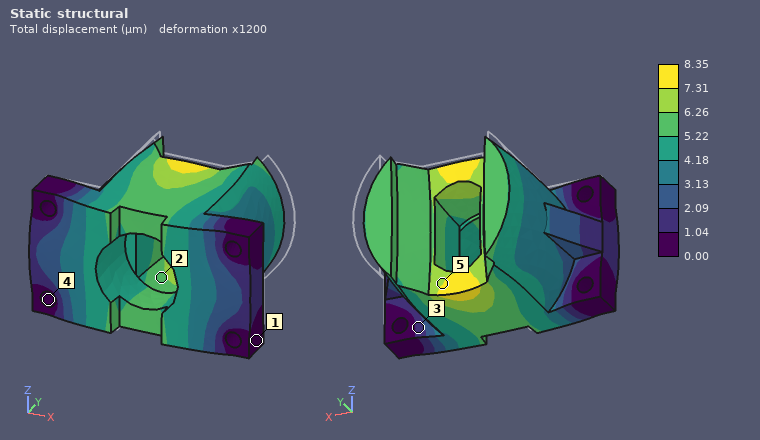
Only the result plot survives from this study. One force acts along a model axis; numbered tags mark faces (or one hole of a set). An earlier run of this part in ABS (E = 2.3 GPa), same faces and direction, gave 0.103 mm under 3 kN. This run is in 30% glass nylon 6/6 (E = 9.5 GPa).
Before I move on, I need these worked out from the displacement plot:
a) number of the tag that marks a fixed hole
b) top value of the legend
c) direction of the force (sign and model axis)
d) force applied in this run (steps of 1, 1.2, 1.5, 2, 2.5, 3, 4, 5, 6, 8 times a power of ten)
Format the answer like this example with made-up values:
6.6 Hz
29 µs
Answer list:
4
8.35 µm
-Y
1 kN
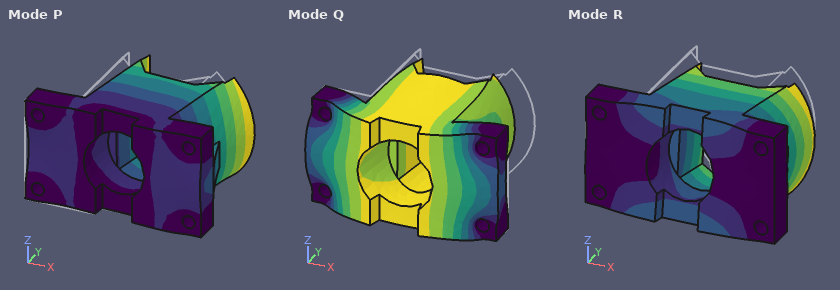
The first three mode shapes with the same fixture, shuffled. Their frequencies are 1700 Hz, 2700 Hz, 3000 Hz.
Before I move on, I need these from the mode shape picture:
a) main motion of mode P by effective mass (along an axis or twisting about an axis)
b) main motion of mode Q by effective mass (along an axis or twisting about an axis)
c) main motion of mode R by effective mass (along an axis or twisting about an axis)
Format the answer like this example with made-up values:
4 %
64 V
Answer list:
along X
along Y
along Z
